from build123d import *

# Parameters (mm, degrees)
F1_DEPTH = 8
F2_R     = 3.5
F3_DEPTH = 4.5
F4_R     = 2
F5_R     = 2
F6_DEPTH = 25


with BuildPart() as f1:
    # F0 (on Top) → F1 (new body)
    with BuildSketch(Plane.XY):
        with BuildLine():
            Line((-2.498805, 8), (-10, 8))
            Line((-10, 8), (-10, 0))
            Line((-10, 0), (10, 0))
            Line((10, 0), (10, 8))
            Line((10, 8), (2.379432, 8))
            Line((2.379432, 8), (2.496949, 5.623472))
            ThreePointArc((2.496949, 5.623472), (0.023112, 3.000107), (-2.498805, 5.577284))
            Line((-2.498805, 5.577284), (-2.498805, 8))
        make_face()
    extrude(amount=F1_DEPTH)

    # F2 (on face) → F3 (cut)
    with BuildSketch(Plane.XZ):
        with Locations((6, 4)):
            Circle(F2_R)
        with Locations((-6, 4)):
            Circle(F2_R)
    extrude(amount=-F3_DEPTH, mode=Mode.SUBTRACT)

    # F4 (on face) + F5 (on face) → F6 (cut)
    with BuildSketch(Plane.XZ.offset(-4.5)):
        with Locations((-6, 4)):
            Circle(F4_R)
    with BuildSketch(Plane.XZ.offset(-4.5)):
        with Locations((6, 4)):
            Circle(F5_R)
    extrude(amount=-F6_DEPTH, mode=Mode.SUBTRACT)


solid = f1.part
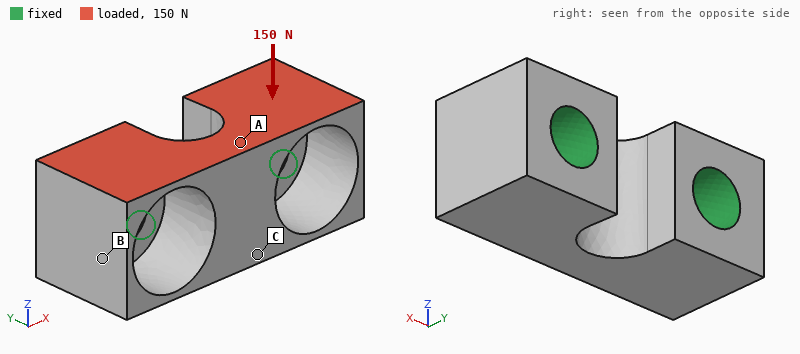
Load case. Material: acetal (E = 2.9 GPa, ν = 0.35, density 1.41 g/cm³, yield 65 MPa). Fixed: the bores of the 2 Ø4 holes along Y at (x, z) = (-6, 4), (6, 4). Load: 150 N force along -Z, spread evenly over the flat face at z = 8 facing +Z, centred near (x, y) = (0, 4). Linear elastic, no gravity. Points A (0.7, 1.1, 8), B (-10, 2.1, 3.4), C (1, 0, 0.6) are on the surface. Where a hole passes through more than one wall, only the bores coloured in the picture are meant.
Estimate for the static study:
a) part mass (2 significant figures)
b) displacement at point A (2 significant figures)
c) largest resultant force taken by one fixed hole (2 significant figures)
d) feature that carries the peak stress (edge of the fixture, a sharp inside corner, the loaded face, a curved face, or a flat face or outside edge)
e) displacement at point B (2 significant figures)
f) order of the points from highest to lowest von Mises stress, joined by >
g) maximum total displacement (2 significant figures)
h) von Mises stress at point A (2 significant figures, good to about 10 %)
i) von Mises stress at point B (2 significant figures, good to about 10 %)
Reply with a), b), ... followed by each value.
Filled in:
a) 0.94 g
b) 24 µm
c) 75 N
d) the loaded face
e) 18 µm
f) B > A > C
g) 57 µm
h) 3.1 MPa
i) 5.6 MPa
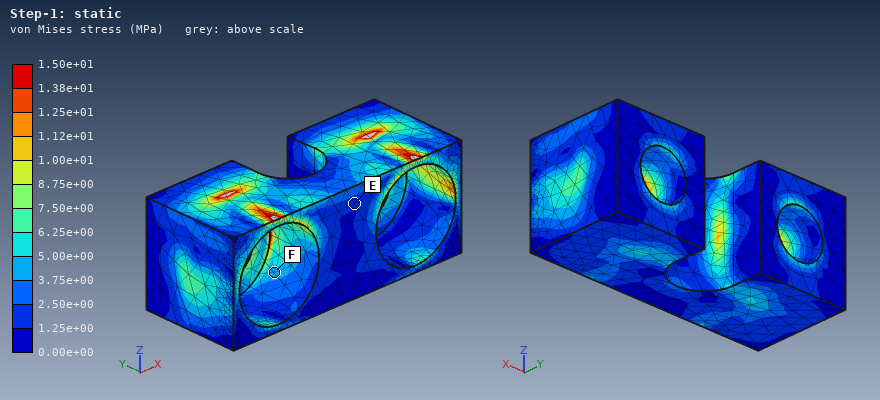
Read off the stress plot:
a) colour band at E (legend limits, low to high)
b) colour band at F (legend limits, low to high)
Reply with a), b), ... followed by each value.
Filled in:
a) 1.25e+00 to 2.50e+00 MPa
b) 3.75e+00 to 5.00e+00 MPa
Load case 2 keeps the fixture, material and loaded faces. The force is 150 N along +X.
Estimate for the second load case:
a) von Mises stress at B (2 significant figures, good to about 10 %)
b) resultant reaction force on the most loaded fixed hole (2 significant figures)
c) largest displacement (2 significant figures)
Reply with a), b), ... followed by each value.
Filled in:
a) 2.5 MPa
b) 79 N
c) 37 µm
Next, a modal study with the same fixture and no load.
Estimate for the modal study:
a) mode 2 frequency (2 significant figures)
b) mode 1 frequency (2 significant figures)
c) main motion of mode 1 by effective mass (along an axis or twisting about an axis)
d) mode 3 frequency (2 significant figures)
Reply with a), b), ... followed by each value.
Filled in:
a) 20 kHz
b) 15 kHz
c) along Z
d) 21 kHz
